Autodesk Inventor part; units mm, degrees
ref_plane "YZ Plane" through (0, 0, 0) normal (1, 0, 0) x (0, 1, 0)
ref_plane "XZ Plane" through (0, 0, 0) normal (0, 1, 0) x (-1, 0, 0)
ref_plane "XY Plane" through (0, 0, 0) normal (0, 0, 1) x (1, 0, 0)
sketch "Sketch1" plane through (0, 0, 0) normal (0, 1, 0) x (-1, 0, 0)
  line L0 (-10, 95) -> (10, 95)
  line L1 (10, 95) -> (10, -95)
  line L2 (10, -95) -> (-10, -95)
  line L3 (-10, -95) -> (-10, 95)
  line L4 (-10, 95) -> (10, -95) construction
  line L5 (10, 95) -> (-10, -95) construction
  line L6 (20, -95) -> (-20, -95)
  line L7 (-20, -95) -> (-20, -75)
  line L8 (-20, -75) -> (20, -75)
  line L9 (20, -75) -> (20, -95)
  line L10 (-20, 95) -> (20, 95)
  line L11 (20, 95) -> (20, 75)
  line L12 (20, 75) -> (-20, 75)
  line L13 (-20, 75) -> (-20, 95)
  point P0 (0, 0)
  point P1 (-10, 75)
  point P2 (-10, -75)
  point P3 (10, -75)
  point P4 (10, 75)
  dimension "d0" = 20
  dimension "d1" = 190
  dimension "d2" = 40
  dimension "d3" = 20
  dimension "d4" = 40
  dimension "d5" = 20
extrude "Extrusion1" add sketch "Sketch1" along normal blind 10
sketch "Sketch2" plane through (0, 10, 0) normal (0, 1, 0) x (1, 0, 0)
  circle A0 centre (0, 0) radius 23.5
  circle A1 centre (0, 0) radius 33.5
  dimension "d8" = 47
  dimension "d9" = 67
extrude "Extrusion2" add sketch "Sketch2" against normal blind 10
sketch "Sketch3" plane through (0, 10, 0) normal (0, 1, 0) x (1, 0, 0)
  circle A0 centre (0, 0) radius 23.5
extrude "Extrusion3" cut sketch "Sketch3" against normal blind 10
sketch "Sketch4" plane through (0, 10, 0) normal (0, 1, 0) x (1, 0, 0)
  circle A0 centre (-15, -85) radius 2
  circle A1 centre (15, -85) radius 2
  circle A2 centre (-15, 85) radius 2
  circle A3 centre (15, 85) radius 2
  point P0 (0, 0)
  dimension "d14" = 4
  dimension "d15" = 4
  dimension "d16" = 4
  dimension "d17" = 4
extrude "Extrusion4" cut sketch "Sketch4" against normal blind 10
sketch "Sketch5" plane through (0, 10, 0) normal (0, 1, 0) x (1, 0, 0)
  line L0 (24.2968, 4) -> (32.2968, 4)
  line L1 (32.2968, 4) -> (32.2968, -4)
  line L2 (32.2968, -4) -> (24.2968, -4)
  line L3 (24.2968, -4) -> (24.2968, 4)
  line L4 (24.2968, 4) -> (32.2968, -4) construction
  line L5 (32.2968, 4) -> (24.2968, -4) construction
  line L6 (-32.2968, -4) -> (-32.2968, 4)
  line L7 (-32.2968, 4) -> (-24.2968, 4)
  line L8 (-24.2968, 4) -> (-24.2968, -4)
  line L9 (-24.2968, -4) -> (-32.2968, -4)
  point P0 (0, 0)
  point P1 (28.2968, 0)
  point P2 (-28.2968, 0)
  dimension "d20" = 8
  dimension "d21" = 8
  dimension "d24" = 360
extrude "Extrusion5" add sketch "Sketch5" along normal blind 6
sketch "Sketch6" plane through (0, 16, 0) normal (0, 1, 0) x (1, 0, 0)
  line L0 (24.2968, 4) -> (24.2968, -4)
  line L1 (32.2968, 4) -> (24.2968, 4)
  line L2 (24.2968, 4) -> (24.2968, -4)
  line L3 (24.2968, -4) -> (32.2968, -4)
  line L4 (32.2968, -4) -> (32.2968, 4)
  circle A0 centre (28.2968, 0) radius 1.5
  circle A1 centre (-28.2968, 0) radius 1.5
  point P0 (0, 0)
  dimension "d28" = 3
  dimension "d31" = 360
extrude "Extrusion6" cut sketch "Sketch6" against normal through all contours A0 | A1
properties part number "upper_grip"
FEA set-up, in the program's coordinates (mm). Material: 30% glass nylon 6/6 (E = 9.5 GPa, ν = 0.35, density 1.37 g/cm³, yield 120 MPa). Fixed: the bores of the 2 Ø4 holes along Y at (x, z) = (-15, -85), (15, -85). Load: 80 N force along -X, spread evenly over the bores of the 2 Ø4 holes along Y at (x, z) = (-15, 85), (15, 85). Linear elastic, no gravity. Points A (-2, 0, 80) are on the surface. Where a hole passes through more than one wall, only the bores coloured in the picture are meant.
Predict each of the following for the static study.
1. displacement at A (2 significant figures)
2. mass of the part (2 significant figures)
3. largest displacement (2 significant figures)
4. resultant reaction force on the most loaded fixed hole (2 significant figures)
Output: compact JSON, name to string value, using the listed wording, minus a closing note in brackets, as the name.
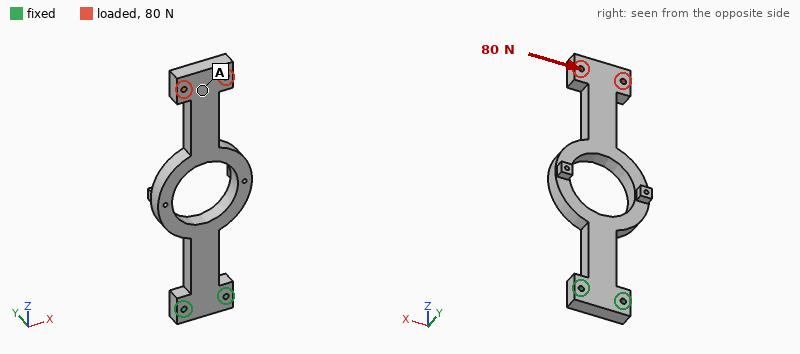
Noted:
{"displacement at A": "1.8 mm", "mass of the part": "70 g", "largest displacement": "2.1 mm", "resultant reaction force on the most loaded fixed hole": "470 N"}
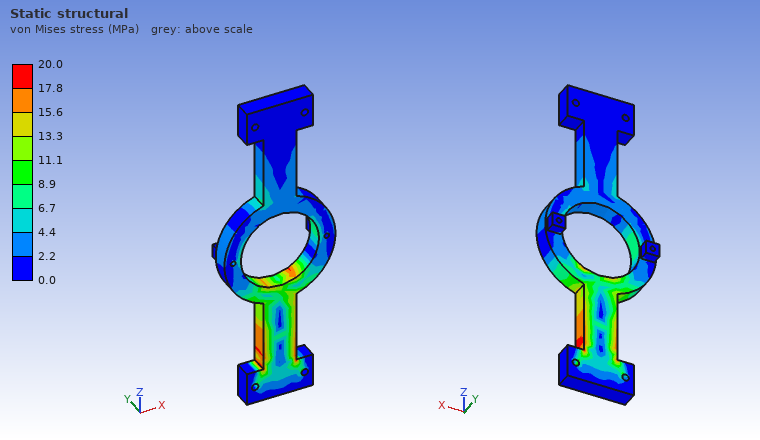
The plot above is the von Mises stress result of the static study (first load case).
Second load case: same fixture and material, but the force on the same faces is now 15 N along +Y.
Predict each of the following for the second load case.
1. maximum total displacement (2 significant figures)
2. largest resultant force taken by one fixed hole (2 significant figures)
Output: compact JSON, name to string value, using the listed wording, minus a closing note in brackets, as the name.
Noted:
{"maximum total displacement": "2.0 mm", "largest resultant force taken by one fixed hole": "7.5 N"}
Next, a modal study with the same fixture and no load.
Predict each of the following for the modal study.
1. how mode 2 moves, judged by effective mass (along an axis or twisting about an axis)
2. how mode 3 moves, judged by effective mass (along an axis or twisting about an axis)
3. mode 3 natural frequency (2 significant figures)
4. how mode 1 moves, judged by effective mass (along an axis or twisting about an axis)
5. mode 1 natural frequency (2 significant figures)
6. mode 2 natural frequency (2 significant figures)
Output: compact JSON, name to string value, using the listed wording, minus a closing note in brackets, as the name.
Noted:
{"how mode 2 moves, judged by effective mass": "along X", "how mode 3 moves, judged by effective mass": "along Y", "mode 3 natural frequency": "600 Hz", "how mode 1 moves, judged by effective mass": "along Y", "mode 1 natural frequency": "100 Hz", "mode 2 natural frequency": "220 Hz"}
